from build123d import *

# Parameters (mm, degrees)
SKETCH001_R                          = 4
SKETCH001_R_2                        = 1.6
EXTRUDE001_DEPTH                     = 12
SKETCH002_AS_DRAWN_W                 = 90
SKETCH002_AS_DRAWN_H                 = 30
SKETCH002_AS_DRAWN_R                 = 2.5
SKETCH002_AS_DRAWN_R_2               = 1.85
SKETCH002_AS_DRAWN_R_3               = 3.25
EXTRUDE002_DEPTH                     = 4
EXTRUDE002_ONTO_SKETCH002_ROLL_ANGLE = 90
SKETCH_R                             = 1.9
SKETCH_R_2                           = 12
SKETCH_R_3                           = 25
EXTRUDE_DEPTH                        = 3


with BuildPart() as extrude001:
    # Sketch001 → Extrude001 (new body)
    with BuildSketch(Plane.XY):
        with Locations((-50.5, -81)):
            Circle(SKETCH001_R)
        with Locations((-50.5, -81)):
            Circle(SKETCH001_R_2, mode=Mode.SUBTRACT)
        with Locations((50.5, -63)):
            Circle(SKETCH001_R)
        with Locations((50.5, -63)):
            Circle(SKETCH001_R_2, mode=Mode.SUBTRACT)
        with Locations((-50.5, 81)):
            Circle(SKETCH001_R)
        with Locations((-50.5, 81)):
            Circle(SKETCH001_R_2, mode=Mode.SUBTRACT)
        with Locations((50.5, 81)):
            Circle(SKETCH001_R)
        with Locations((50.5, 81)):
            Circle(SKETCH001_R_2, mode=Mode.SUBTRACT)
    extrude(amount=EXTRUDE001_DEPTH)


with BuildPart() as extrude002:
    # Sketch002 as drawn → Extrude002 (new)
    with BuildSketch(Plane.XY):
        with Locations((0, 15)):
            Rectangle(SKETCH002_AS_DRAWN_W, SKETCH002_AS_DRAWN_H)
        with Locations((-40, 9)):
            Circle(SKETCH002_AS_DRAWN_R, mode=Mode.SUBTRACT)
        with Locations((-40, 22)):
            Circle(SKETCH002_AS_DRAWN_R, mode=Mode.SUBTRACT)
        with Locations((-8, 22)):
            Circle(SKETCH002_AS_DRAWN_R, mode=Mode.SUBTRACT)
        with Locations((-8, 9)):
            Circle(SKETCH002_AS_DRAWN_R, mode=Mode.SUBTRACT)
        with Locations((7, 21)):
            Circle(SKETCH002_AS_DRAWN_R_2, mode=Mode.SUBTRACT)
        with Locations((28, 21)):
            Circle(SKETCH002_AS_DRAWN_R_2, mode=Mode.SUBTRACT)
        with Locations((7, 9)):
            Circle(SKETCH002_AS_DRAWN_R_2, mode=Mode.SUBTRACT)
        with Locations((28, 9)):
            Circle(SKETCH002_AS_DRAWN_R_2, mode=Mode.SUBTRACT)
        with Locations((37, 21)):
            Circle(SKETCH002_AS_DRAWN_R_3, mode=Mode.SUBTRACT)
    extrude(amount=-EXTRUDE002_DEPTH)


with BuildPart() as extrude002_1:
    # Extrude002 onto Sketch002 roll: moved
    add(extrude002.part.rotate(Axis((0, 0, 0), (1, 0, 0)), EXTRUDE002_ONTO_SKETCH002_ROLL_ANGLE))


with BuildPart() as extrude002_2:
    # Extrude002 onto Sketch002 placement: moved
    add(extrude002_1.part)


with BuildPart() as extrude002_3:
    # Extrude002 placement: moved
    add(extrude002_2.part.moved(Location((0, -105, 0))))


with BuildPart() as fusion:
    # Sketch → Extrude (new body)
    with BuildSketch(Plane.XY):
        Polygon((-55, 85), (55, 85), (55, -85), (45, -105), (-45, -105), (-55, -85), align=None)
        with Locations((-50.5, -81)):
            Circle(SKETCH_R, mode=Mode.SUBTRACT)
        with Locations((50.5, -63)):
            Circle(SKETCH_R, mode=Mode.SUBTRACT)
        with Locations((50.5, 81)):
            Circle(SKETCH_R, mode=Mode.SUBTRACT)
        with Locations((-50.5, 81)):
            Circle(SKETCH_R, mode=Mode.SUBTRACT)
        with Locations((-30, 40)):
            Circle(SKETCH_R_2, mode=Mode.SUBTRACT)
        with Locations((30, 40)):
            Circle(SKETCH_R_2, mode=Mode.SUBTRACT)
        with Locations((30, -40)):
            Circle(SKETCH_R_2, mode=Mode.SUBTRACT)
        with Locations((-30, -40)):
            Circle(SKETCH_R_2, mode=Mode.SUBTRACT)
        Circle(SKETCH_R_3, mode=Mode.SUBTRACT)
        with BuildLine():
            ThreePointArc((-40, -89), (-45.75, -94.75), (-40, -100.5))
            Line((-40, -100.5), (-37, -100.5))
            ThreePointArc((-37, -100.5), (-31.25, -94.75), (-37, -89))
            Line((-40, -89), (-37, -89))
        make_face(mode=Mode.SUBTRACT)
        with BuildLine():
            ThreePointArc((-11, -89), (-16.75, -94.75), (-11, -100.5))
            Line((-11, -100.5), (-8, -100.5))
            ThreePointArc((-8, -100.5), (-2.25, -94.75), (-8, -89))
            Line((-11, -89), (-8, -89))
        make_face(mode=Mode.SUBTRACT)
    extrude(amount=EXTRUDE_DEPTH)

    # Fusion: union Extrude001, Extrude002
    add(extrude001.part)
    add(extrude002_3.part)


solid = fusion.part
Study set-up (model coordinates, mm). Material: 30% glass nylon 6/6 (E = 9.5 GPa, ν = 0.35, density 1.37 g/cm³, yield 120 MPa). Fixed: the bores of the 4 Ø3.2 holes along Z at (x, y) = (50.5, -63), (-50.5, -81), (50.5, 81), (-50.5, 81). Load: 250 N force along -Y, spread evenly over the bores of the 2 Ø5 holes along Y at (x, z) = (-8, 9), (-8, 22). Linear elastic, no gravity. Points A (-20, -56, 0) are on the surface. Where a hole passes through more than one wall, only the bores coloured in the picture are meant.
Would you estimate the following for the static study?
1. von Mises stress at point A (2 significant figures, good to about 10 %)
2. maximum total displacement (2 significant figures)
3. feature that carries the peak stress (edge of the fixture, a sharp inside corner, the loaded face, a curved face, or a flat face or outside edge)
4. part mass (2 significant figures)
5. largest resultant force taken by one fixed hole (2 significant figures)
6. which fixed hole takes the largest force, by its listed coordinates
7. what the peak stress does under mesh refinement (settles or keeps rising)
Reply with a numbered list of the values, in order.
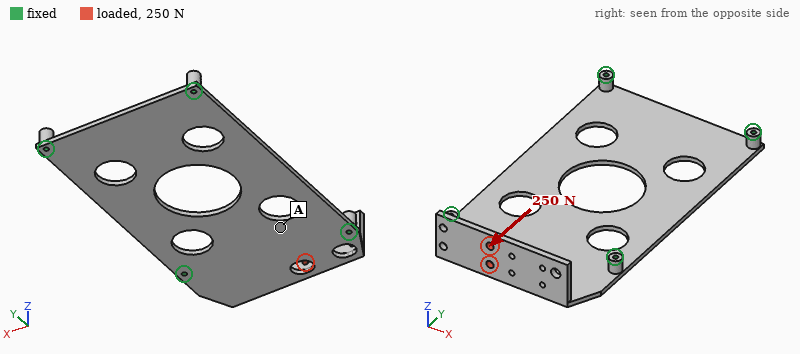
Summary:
1. 6.5 MPa
2. 2.5 mm
3. a sharp inside corner
4. 83 g
5. 120 N
6. (-50.5, -81)
7. keeps rising
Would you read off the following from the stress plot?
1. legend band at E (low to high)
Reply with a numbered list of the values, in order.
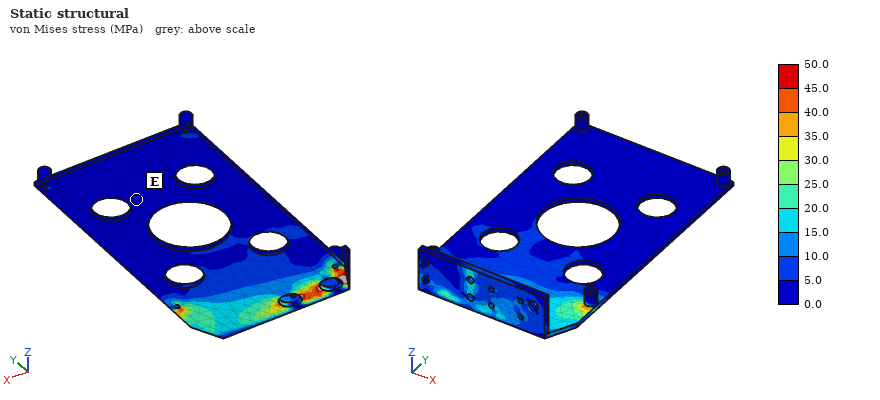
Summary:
1. 0.0 to 5.0 MPa
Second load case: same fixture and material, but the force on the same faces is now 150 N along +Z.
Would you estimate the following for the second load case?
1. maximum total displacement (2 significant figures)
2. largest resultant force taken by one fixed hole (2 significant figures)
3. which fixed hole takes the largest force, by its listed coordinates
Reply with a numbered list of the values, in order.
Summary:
1. 2.2 mm
2. 97 N
3. (-50.5, -81)
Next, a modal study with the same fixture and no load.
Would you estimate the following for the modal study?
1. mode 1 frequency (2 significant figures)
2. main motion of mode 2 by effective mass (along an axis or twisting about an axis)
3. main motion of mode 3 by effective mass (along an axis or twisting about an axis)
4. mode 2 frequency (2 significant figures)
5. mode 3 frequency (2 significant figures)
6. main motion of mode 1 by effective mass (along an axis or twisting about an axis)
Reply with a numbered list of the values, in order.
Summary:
1. 280 Hz
2. along Z
3. twisting about Y
4. 370 Hz
5. 450 Hz
6. along Z
